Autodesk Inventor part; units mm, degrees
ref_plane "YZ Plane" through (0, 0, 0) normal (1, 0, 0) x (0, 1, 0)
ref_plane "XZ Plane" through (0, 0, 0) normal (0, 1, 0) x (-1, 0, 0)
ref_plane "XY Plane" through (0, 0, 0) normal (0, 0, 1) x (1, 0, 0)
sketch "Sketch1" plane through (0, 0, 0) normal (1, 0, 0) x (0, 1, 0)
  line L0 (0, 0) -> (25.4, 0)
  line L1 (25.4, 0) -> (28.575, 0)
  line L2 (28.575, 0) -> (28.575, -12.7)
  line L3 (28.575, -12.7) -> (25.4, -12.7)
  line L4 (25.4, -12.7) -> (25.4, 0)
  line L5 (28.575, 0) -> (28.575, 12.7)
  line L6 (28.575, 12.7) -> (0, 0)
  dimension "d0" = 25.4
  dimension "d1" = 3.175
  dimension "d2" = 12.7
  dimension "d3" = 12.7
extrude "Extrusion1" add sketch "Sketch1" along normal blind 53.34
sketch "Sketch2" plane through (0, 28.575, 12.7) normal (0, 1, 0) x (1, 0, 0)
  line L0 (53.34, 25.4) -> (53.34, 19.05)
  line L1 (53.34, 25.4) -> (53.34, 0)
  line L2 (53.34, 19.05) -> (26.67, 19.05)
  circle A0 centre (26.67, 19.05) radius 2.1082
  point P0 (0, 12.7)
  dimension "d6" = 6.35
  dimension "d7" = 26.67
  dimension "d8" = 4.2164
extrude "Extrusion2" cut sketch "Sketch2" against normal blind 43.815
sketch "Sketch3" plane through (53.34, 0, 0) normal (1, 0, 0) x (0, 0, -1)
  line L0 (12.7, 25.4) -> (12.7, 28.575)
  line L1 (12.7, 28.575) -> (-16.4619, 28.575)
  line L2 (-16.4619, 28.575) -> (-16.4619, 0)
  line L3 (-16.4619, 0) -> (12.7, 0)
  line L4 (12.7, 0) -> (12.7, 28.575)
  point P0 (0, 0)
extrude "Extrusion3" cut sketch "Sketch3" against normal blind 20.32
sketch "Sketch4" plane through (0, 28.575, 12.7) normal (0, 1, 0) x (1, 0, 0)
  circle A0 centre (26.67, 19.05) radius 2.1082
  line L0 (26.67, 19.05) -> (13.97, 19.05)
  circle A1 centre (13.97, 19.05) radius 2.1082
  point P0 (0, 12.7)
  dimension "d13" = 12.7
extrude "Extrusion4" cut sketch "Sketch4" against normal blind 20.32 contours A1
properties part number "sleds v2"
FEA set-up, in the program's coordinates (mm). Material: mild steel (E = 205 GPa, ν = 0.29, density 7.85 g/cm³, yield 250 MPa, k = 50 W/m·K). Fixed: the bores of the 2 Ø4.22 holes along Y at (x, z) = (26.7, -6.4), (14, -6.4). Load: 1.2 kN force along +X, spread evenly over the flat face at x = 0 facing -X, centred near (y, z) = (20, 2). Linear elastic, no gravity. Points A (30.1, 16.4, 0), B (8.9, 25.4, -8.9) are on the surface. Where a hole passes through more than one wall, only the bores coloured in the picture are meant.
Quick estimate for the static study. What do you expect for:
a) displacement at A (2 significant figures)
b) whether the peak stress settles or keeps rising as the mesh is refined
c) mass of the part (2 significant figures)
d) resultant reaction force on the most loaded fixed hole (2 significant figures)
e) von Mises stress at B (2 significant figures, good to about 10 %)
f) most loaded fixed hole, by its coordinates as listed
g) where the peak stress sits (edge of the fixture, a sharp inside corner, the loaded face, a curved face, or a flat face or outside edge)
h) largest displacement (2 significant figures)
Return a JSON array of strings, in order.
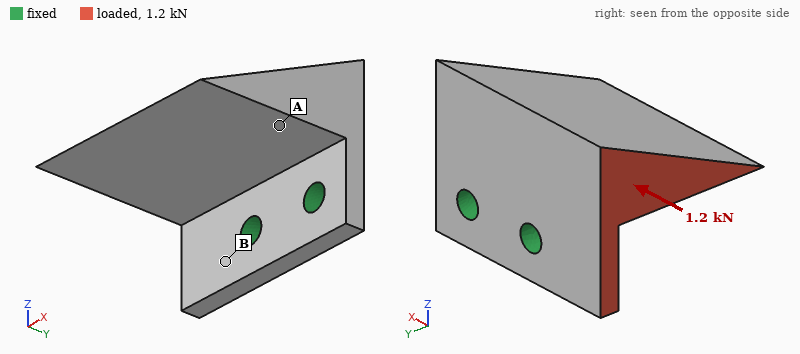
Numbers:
["8.1 µm", "keeps rising", "57 g", "1.0 kN", "27 MPa", "(14, -6.4)", "edge of the fixture", "18 µm"]
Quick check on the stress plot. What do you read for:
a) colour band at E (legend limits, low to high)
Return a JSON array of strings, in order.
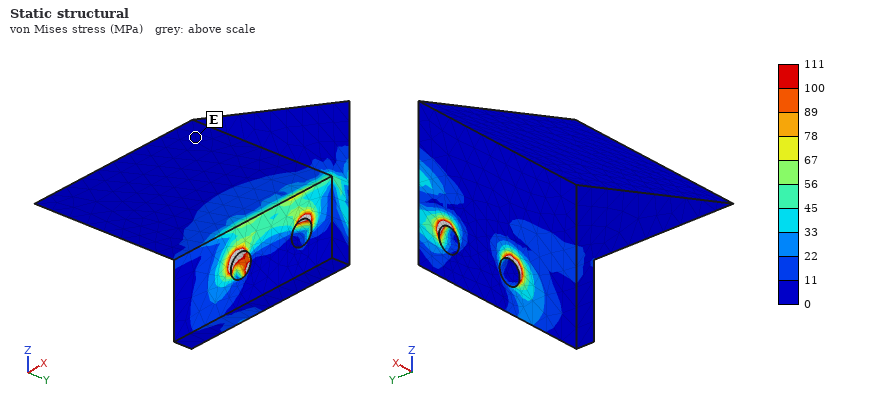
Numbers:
["0 to 11 MPa"]
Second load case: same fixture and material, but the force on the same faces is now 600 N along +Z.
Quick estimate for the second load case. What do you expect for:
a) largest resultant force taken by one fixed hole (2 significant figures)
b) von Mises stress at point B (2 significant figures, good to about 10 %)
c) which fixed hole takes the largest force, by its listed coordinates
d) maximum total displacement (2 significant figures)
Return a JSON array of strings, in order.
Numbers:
["1.0 kN", "39 MPa", "(14, -6.4)", "55 µm"]
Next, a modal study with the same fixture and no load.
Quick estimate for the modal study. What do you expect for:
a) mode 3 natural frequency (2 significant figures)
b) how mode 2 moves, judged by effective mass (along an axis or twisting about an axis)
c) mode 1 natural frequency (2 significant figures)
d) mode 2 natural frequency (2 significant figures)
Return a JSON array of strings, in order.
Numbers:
["13 kHz", "along X", "2800 Hz", "6200 Hz"]
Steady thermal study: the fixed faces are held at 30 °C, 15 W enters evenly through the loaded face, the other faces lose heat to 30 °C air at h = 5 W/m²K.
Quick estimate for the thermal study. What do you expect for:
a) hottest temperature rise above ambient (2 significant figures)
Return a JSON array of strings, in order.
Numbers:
["47 K"]
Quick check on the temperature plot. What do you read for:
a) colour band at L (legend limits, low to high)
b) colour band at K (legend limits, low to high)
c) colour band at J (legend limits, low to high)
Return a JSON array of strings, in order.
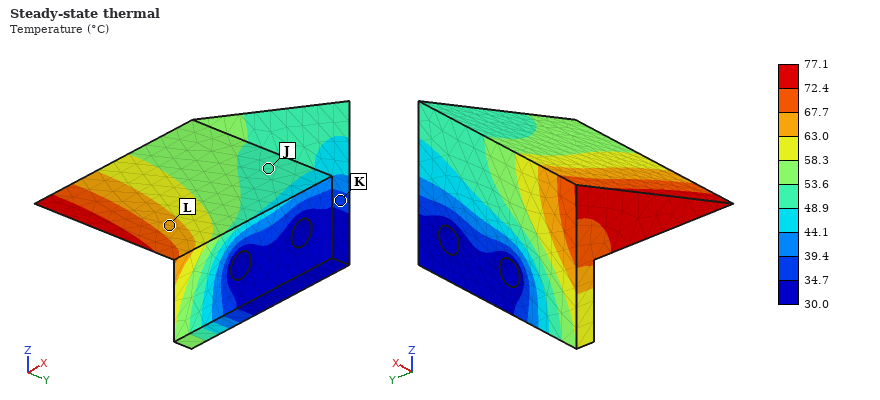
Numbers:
["63.0 to 67.7 °C", "34.7 to 39.4 °C", "48.9 to 53.6 °C"]
